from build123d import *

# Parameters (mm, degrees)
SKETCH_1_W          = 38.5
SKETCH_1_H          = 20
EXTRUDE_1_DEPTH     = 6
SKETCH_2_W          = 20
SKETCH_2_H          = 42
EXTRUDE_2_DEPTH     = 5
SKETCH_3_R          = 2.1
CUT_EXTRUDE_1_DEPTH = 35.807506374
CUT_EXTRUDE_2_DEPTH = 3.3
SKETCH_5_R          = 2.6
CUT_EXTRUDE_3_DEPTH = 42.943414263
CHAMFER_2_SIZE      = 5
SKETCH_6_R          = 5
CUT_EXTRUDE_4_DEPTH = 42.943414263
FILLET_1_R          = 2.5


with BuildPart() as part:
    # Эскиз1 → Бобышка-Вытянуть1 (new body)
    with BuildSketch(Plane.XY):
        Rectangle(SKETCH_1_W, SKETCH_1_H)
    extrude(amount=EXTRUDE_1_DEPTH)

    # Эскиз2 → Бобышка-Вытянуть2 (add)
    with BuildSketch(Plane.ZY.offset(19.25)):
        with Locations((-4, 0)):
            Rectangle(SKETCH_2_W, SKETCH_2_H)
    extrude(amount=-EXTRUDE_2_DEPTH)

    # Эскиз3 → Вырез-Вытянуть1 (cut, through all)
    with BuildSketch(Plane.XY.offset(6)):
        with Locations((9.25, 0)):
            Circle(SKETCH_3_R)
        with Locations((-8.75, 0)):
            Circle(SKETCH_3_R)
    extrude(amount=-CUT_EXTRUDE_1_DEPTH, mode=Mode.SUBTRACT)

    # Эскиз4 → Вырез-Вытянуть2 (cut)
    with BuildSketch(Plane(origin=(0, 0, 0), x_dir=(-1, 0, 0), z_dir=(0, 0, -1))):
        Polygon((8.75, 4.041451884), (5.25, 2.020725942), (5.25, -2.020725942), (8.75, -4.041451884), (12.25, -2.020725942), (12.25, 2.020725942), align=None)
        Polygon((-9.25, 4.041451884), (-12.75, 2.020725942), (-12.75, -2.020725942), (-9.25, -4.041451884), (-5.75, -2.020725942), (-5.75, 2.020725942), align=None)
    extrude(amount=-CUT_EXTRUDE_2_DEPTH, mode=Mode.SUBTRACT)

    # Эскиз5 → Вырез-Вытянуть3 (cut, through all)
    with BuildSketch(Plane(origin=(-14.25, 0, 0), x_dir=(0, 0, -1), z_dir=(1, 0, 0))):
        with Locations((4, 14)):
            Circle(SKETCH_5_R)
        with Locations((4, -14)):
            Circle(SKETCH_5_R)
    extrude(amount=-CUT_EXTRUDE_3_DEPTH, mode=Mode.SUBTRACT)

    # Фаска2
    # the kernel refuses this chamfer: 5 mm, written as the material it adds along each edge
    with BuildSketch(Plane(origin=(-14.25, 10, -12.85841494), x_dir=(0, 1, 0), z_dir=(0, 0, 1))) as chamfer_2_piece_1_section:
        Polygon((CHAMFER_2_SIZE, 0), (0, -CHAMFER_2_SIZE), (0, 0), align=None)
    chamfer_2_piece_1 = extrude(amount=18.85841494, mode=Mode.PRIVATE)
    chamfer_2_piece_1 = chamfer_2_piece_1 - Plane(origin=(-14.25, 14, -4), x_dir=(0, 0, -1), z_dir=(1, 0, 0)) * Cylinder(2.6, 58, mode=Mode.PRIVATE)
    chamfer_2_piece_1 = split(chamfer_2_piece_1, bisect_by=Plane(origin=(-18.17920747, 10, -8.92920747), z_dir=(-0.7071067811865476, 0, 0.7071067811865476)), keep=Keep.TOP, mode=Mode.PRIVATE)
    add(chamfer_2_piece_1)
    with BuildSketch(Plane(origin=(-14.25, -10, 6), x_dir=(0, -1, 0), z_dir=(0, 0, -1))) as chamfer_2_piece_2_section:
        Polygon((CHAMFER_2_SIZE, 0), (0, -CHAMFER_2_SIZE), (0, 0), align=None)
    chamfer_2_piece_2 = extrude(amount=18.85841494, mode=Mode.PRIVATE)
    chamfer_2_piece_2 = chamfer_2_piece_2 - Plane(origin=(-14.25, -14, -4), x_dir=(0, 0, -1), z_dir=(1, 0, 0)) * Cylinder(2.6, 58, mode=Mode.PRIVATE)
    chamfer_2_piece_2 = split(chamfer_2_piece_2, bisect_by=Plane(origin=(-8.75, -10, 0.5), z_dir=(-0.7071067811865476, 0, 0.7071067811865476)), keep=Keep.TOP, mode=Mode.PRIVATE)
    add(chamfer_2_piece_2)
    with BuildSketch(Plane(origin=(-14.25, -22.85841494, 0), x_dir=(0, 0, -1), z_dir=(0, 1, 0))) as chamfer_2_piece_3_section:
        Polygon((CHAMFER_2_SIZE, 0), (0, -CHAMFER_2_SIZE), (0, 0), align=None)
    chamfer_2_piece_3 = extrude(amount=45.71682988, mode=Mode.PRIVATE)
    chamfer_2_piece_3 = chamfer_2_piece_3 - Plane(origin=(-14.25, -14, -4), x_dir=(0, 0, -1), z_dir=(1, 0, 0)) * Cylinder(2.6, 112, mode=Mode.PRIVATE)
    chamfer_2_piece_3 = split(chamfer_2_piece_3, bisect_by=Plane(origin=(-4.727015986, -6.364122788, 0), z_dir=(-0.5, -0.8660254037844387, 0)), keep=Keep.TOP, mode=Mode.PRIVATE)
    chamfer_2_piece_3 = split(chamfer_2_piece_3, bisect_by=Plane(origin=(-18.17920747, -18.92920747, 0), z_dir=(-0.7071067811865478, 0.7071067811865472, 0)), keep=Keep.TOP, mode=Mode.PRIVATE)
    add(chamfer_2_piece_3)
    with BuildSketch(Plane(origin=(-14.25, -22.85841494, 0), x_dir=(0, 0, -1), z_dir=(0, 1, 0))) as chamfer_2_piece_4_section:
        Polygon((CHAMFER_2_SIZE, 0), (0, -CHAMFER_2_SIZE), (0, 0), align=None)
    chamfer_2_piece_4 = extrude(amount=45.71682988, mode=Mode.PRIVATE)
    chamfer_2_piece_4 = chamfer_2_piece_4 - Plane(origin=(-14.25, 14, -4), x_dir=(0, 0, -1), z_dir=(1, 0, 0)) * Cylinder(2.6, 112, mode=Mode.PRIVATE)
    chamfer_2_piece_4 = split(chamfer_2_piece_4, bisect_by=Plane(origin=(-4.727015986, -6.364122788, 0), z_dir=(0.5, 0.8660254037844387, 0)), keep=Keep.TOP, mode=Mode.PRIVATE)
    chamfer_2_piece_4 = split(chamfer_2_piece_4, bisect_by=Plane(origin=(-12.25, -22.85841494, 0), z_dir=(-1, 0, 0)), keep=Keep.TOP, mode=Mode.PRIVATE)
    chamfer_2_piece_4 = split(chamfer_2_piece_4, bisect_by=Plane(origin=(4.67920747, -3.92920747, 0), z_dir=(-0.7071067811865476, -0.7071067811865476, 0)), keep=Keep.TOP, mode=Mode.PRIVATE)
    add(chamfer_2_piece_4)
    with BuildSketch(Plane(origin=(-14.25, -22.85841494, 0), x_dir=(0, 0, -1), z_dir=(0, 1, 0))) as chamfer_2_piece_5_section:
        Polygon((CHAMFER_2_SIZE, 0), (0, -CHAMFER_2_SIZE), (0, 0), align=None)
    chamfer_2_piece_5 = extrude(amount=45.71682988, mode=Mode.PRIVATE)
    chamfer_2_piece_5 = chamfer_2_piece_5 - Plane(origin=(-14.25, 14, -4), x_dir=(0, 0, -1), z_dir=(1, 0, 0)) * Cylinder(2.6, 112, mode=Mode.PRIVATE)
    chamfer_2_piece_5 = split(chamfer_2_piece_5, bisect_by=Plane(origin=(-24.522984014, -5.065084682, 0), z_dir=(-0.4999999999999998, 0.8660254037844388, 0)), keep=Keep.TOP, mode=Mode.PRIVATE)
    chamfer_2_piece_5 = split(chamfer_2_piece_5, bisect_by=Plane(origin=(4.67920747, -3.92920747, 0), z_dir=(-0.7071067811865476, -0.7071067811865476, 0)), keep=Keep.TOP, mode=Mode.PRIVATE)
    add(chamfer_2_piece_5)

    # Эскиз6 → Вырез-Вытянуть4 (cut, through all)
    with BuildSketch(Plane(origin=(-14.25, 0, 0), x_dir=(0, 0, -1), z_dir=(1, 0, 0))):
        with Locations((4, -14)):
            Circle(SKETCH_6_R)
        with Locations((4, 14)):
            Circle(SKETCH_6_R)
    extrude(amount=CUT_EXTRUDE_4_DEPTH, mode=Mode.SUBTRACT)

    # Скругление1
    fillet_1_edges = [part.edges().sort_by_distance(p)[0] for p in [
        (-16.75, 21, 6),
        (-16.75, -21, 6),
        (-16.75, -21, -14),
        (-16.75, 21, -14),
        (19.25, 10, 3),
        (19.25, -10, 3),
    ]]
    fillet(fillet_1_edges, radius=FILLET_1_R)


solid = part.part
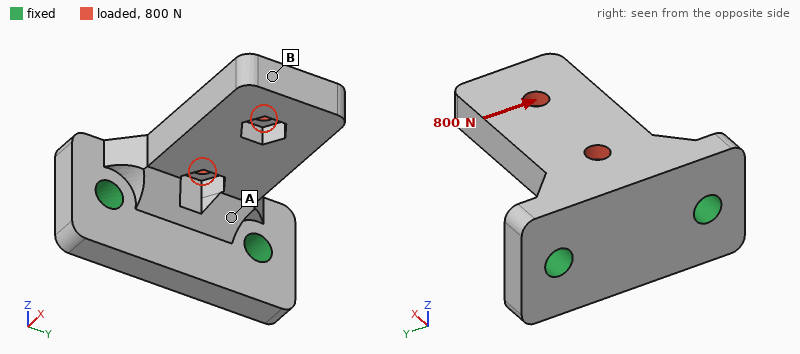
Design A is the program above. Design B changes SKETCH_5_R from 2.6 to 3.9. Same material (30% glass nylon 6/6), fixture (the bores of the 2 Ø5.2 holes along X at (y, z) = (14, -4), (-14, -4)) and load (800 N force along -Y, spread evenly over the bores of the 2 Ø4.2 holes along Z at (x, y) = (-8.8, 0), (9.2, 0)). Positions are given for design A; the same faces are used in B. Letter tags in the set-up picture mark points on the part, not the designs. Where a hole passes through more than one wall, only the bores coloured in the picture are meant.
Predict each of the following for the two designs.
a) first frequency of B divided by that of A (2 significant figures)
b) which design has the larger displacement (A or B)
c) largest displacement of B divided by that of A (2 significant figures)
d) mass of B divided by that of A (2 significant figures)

1.1
A
0.85
0.97
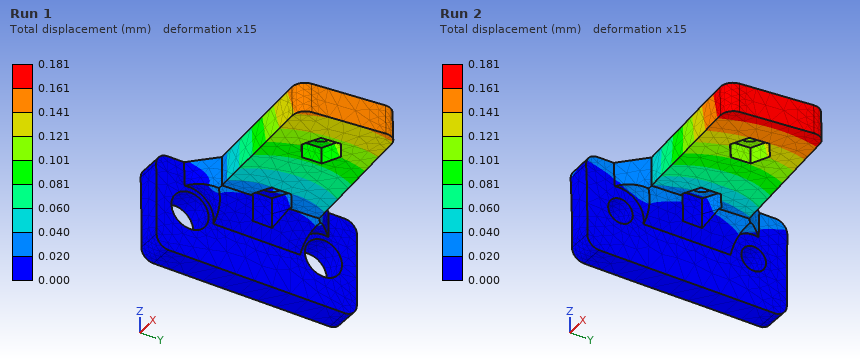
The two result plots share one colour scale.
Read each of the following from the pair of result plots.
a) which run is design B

Run 1
